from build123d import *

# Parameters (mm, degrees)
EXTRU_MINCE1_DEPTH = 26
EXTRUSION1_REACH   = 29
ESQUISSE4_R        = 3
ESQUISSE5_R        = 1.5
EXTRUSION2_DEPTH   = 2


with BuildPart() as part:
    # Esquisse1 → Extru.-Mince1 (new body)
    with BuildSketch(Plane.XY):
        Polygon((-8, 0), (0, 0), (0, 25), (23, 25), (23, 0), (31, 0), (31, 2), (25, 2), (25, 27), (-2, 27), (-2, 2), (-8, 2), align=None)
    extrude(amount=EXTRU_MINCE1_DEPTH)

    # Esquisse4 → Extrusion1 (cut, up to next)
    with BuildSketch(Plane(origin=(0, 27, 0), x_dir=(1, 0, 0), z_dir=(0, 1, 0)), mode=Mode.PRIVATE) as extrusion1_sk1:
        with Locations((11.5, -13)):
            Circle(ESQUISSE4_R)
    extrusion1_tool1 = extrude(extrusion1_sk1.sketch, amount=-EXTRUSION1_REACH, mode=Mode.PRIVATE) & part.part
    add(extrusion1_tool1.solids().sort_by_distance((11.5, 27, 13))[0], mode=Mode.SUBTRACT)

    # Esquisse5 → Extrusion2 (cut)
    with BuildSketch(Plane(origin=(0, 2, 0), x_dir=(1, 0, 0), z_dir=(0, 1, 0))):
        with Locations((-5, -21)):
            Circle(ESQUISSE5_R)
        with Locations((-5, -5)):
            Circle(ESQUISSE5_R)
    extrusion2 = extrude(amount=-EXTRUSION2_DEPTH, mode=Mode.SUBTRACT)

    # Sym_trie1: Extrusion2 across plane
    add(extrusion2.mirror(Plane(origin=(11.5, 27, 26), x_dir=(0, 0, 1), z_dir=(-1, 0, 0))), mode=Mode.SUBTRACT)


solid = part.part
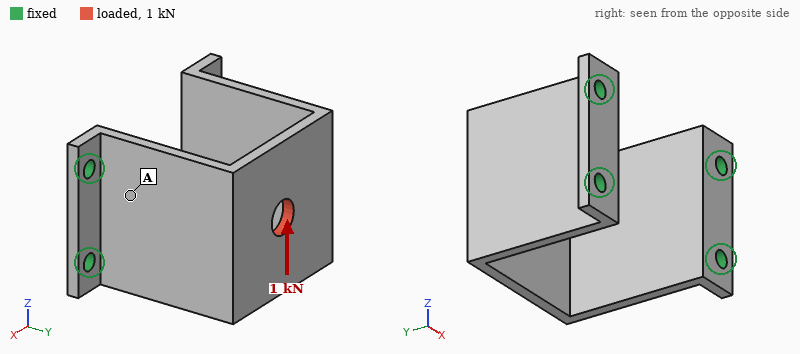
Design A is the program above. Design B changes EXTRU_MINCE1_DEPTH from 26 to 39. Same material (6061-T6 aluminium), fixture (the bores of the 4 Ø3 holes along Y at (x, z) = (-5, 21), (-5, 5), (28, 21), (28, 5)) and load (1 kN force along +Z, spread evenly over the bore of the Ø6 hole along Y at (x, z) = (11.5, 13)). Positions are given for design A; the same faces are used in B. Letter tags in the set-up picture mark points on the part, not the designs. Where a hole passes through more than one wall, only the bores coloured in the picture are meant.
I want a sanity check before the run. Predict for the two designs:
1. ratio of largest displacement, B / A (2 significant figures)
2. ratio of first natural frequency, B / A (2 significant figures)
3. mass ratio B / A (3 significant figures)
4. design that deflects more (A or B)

1.1
0.94
1.51
B
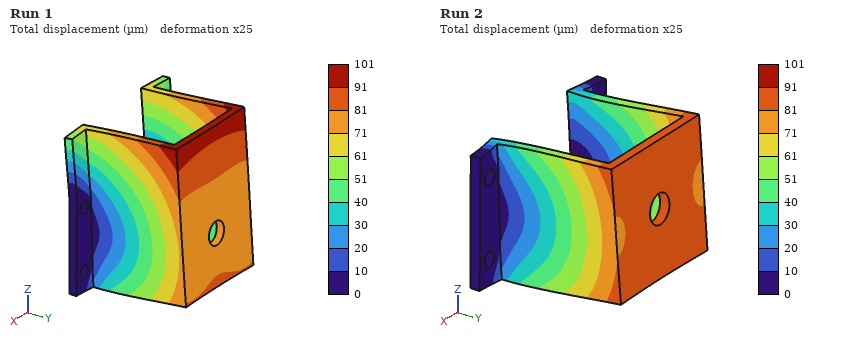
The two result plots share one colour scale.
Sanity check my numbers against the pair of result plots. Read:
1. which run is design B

Run 1
